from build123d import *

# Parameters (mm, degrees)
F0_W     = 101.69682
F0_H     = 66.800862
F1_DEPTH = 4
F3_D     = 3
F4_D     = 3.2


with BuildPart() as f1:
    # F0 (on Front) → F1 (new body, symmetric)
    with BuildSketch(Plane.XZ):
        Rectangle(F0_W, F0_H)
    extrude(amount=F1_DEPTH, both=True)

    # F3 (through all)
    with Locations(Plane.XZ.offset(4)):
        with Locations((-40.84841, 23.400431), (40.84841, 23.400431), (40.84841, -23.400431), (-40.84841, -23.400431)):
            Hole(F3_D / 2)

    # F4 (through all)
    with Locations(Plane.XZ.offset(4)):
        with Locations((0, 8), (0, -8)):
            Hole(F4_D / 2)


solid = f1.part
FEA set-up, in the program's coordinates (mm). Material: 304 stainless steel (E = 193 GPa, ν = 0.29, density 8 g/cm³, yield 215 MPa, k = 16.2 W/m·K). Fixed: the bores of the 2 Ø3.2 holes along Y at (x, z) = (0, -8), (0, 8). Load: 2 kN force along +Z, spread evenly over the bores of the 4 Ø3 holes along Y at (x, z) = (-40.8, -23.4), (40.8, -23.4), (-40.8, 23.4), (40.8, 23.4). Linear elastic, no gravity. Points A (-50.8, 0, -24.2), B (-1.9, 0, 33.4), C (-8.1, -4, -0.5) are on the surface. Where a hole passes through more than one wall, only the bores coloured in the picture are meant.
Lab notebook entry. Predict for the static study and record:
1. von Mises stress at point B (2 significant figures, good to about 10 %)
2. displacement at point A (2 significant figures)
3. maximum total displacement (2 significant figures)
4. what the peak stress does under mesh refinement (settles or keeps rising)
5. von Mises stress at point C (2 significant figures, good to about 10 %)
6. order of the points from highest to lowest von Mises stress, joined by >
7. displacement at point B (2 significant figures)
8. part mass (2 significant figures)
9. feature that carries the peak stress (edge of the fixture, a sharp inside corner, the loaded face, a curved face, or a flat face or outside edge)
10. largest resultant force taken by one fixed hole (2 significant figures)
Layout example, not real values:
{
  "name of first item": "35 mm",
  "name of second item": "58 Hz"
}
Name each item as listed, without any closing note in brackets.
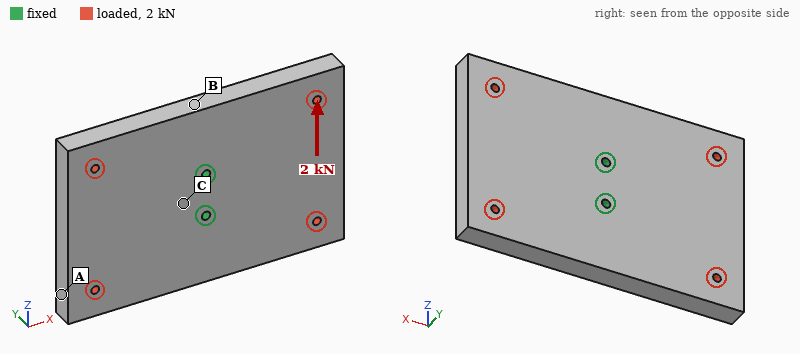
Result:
{
  "von Mises stress at point B": "8.0 MPa",
  "displacement at point A": "2.4 µm",
  "maximum total displacement": "2.5 µm",
  "what the peak stress does under mesh refinement": "keeps rising",
  "von Mises stress at point C": "5.7 MPa",
  "order of the points from highest to lowest von Mises stress, joined by >": "B > C > A",
  "displacement at point B": "0.53 µm",
  "part mass": "430 g",
  "feature that carries the peak stress": "edge of the fixture",
  "largest resultant force taken by one fixed hole": "1.0 kN"
}
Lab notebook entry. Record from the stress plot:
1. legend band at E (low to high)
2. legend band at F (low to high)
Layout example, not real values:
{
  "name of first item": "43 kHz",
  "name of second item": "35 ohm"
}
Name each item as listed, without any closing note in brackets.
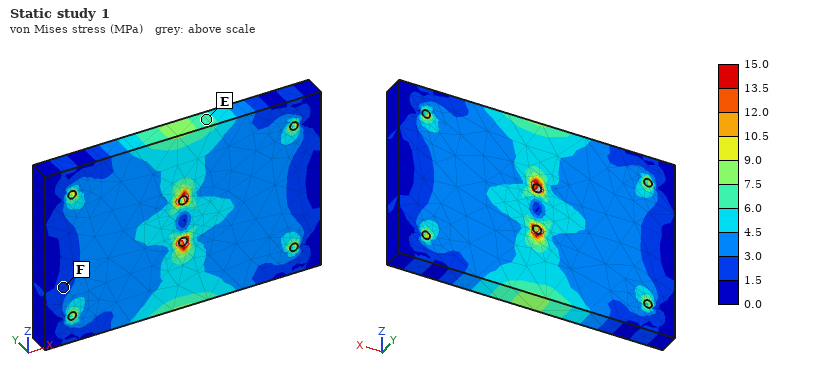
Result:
{
  "legend band at E": "6.0 to 7.5 MPa",
  "legend band at F": "1.5 to 3.0 MPa"
}
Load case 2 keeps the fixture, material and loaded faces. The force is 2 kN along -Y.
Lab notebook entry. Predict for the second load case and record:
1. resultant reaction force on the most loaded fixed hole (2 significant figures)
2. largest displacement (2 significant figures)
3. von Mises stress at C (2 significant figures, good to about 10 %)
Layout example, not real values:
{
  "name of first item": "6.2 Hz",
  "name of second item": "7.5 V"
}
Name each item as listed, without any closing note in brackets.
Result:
{
  "resultant reaction force on the most loaded fixed hole": "1.0 kN",
  "largest displacement": "56 µm",
  "von Mises stress at C": "42 MPa"
}
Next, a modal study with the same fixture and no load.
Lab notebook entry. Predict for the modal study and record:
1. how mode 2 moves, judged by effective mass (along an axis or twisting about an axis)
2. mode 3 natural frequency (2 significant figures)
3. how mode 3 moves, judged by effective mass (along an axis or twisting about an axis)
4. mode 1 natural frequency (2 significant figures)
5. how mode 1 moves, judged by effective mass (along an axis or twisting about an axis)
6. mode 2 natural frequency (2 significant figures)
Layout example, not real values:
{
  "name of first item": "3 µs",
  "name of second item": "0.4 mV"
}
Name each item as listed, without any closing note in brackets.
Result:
{
  "how mode 2 moves, judged by effective mass": "along Y",
  "mode 3 natural frequency": "3500 Hz",
  "how mode 3 moves, judged by effective mass": "twisting about X",
  "mode 1 natural frequency": "1700 Hz",
  "how mode 1 moves, judged by effective mass": "twisting about Z",
  "mode 2 natural frequency": "2500 Hz"
}
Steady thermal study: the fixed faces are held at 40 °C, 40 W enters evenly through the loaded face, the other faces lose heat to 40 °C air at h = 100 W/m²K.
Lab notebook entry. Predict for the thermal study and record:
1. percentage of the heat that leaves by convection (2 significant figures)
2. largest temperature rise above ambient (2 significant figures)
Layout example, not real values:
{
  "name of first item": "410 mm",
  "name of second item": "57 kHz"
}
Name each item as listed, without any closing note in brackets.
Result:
{
  "percentage of the heat that leaves by convection": "86 %",
  "largest temperature rise above ambient": "57 K"
}
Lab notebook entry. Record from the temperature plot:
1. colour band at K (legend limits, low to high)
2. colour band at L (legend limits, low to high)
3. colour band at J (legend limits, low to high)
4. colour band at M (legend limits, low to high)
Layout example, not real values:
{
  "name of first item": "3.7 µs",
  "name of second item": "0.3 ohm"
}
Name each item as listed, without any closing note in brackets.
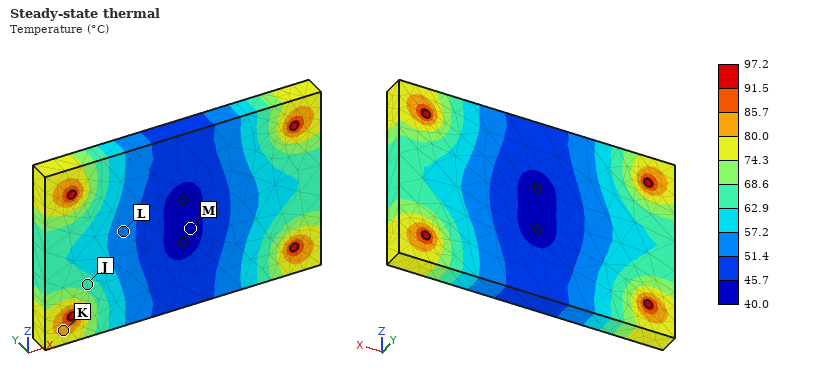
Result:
{
  "colour band at K": "80.0 to 85.7 °C",
  "colour band at L": "51.4 to 57.2 °C",
  "colour band at J": "62.9 to 68.6 °C",
  "colour band at M": "40.0 to 45.7 °C"
}
